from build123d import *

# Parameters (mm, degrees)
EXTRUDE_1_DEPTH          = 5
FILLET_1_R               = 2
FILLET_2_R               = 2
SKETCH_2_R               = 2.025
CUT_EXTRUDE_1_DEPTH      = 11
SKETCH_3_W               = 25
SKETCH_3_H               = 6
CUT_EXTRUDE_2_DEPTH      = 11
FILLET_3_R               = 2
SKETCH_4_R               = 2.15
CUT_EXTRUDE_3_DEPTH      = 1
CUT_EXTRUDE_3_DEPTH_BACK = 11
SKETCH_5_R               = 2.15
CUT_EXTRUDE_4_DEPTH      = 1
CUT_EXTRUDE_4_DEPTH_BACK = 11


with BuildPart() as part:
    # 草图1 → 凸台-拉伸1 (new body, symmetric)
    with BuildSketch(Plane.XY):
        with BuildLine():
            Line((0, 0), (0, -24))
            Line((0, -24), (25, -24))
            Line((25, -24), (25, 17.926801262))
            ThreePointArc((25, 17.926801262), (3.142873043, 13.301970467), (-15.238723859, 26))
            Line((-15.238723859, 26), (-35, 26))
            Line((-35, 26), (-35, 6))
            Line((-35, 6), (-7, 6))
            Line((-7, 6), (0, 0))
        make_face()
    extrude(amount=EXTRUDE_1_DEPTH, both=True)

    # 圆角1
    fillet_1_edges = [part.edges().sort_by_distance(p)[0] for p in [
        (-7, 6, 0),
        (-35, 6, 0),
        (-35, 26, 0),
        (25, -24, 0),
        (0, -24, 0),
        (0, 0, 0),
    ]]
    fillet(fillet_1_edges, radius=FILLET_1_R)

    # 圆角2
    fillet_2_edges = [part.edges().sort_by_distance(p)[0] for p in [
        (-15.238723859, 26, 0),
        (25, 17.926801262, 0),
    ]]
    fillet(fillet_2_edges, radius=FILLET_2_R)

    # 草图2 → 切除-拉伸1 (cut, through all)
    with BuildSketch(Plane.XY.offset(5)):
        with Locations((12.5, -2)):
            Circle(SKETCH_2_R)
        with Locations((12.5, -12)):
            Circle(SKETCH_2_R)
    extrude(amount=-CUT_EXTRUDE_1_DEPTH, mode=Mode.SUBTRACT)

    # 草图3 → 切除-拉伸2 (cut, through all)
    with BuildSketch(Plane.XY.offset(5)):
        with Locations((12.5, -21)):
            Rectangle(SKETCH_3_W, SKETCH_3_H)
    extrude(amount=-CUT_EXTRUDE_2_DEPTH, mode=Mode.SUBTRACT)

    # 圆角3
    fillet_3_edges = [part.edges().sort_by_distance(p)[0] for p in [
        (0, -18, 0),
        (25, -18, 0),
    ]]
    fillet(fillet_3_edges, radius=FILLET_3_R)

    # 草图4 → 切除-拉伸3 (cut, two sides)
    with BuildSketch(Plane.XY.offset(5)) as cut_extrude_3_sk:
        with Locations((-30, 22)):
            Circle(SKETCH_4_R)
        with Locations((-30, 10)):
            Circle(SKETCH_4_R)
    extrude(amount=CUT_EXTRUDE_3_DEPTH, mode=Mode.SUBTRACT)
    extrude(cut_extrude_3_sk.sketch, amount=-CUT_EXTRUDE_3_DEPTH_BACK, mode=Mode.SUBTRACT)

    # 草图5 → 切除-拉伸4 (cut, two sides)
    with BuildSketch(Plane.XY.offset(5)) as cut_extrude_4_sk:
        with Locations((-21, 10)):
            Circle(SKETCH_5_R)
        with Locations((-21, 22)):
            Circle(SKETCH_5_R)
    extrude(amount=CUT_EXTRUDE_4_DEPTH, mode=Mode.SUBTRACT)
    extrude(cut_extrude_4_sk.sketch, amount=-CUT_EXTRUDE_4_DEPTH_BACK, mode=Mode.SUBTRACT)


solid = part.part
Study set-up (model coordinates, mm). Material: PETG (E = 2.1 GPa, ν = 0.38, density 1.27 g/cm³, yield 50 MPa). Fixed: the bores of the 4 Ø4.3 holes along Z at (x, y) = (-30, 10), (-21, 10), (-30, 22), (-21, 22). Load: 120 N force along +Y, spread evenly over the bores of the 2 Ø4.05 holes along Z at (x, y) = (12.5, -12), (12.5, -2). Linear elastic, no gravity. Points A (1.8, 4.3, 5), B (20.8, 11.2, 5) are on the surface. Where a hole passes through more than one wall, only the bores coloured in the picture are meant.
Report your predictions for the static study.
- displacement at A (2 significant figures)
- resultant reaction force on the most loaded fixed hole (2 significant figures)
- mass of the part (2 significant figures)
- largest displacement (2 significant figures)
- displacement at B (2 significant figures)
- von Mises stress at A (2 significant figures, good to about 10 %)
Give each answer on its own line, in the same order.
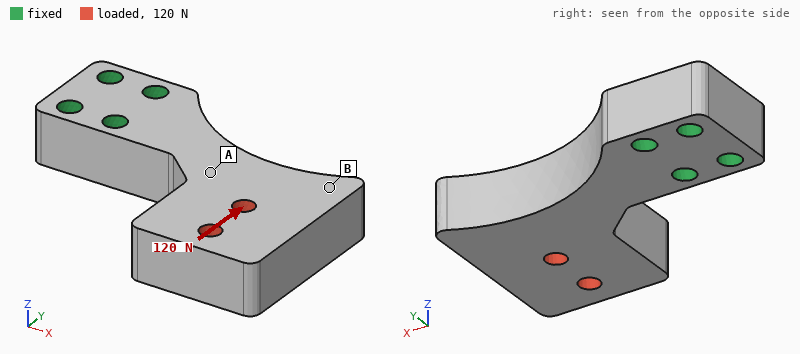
0.20 mm
300 N
17 g
0.75 mm
0.50 mm
3.2 MPa
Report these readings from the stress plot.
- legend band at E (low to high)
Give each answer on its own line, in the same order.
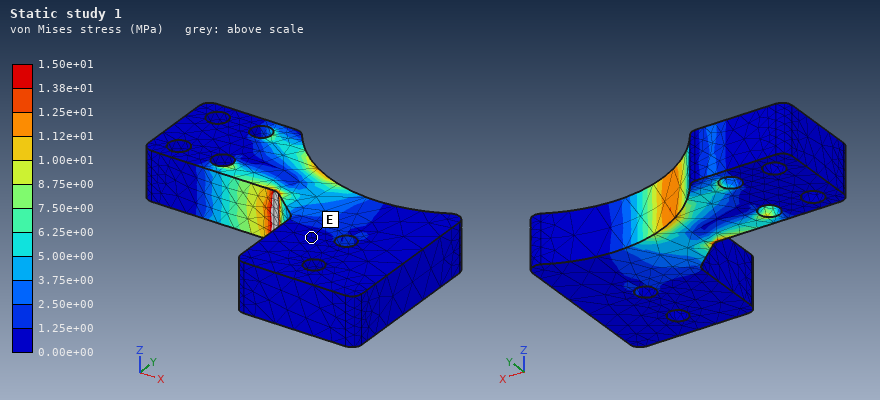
0.00e+00 to 1.25e+00 MPa
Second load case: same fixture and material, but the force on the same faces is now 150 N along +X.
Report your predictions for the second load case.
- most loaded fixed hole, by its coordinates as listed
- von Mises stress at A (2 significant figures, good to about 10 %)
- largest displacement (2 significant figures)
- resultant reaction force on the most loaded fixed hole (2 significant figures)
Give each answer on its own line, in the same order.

(-21, 10)
4.3 MPa
0.88 mm
320 N
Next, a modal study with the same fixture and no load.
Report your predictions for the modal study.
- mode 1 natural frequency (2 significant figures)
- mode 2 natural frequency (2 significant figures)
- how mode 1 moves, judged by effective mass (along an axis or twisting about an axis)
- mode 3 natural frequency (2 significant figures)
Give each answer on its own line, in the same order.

570 Hz
700 Hz
along Z
1300 Hz
